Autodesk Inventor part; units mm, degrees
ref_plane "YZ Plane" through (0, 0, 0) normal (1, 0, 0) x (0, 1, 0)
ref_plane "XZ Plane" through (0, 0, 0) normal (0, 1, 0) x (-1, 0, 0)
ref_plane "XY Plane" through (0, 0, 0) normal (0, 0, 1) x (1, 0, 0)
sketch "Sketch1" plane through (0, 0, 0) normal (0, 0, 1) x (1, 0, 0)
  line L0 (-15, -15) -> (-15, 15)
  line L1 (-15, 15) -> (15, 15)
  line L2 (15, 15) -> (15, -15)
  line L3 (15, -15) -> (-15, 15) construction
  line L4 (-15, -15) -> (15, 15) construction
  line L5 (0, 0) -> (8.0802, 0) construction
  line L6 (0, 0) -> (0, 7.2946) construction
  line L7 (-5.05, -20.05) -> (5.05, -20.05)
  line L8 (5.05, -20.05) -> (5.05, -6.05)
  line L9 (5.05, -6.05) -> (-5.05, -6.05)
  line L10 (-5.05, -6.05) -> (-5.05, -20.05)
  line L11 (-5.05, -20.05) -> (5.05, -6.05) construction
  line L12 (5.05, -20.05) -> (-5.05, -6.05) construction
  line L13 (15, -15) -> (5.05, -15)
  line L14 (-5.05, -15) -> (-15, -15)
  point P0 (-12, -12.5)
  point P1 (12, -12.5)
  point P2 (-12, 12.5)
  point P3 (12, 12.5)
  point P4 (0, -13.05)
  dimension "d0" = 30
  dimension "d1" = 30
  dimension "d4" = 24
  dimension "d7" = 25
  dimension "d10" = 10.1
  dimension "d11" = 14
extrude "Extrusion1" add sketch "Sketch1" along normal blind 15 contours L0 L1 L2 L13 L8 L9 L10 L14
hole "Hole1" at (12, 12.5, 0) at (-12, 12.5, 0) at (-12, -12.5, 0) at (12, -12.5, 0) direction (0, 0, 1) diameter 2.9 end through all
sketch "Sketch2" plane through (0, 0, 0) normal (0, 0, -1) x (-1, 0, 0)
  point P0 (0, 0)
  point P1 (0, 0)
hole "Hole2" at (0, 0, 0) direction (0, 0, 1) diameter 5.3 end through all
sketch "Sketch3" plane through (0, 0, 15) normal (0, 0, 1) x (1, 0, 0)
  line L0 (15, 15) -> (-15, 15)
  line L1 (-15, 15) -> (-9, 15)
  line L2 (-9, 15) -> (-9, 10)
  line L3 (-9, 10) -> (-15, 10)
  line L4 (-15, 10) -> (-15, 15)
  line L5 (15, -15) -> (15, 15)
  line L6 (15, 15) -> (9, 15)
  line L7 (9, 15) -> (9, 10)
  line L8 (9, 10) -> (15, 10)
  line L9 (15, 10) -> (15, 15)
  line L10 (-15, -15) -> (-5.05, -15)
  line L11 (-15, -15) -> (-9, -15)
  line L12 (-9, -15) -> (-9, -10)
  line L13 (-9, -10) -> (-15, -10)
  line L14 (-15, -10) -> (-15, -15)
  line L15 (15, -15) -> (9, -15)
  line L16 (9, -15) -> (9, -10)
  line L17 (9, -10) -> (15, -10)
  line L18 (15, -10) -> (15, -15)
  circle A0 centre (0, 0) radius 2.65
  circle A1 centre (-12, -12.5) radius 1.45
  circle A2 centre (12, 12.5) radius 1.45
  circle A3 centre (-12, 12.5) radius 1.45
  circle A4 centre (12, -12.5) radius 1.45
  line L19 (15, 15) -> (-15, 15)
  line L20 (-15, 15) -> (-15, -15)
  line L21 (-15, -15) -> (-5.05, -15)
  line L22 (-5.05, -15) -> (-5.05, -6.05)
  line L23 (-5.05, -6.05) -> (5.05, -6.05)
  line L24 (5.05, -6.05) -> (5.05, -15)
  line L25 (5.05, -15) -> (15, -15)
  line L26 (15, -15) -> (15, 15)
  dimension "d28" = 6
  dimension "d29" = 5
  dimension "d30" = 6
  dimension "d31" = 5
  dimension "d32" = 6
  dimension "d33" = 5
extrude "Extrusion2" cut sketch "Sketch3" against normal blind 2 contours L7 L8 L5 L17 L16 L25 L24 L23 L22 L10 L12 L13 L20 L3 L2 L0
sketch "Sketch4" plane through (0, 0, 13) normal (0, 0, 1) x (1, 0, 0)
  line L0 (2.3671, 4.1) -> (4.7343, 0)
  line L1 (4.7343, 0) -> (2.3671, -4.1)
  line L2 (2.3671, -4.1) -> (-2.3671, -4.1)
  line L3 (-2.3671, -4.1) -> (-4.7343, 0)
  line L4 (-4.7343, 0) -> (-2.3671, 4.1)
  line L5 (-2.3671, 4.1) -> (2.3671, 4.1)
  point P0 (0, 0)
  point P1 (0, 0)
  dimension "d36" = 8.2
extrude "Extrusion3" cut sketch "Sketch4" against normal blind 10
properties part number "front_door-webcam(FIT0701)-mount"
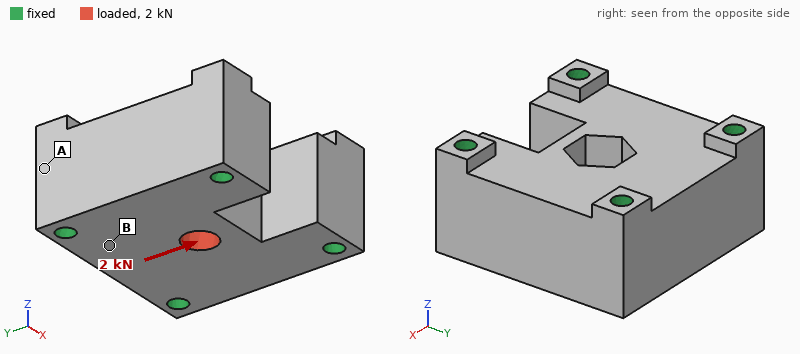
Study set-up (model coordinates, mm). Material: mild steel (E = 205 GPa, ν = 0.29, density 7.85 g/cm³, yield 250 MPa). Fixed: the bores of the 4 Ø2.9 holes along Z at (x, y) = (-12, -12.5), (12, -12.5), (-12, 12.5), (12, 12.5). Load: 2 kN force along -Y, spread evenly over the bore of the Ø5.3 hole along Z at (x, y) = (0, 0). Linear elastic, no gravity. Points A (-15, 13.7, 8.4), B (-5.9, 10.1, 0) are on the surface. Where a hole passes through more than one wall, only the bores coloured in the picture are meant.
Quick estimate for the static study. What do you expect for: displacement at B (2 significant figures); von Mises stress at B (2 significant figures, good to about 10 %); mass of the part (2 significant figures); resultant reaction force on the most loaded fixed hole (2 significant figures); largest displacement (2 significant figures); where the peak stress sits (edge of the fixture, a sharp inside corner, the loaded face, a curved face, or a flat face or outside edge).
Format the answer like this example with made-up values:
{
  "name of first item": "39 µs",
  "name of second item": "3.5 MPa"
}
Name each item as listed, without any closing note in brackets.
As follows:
{
  "displacement at B": "0.47 µm",
  "von Mises stress at B": "12 MPa",
  "mass of the part": "76 g",
  "resultant reaction force on the most loaded fixed hole": "640 N",
  "largest displacement": "2.6 µm",
  "where the peak stress sits": "a sharp inside corner"
}
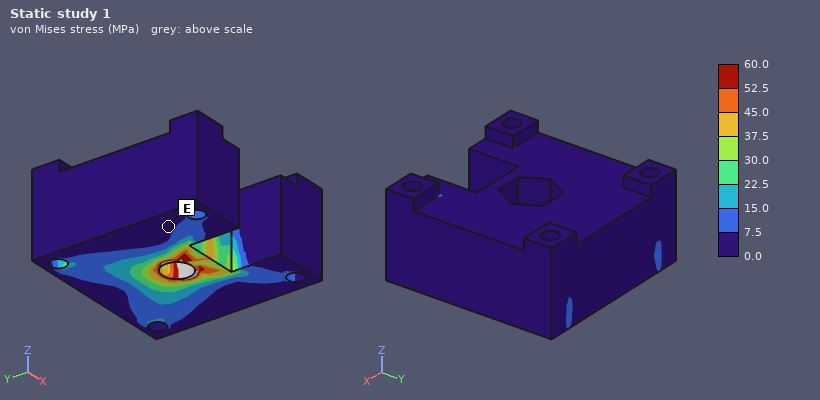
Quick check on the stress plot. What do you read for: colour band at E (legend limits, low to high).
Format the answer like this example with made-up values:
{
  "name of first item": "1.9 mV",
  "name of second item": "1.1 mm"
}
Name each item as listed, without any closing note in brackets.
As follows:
{
  "colour band at E": "0.0 to 7.5 MPa"
}
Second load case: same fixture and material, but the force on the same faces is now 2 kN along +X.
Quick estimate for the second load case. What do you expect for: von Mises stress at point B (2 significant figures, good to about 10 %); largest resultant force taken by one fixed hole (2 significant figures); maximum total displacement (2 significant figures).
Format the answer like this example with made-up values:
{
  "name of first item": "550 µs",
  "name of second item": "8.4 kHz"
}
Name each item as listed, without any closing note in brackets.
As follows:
{
  "von Mises stress at point B": "9.1 MPa",
  "largest resultant force taken by one fixed hole": "780 N",
  "maximum total displacement": "1.7 µm"
}
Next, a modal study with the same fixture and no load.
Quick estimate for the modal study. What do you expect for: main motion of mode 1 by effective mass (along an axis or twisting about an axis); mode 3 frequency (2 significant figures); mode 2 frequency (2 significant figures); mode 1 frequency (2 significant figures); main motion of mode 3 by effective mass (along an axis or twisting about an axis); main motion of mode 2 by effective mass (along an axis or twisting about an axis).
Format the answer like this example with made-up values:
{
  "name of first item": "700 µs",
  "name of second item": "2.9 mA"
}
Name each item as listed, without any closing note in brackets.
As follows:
{
  "main motion of mode 1 by effective mass": "along Z",
  "mode 3 frequency": "55 kHz",
  "mode 2 frequency": "47 kHz",
  "mode 1 frequency": "43 kHz",
  "main motion of mode 3 by effective mass": "twisting about Y",
  "main motion of mode 2 by effective mass": "along X"
}
